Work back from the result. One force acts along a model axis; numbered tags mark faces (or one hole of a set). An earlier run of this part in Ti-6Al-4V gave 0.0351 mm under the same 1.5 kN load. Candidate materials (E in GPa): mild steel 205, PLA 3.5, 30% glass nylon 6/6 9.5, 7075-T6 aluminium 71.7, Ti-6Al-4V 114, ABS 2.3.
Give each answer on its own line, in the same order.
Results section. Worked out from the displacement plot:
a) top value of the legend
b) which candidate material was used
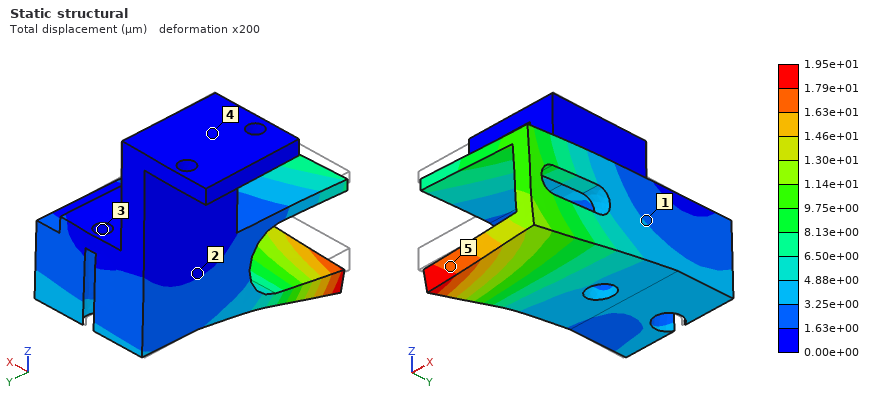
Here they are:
1.95e+01 µm
mild steel
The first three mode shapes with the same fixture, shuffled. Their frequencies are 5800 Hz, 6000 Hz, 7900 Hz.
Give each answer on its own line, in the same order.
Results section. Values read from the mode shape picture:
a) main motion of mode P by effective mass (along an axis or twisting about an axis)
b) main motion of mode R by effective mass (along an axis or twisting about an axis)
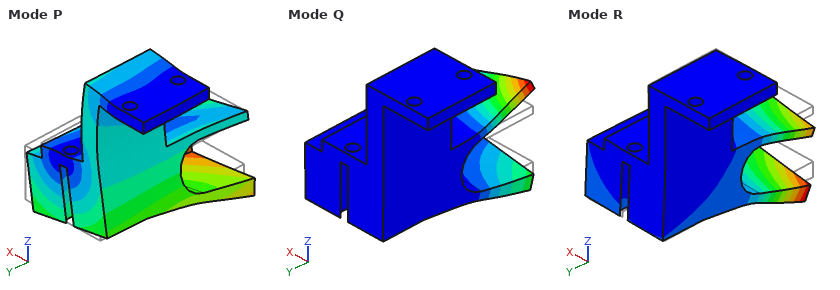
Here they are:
along X
along Z
